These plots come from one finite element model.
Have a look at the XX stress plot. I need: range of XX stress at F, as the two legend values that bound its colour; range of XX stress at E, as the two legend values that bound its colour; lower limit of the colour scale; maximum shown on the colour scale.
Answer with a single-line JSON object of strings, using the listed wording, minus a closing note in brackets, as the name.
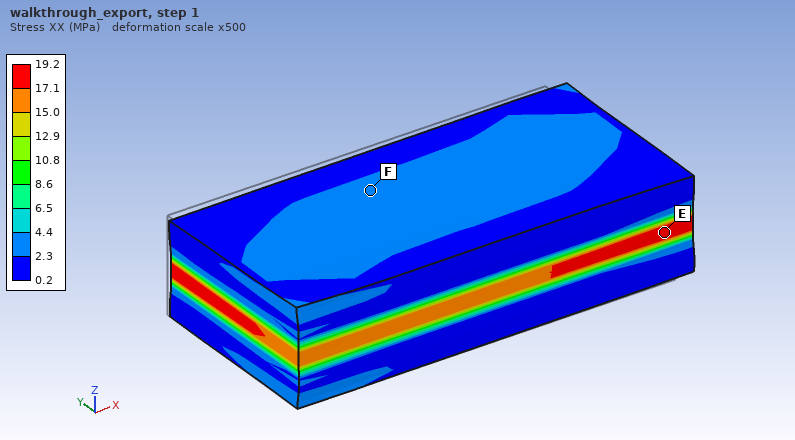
{"range of XX stress at F, as the two legend values that bound its colour": "2.3 to 4.4 MPa", "range of XX stress at E, as the two legend values that bound its colour": "17.1 to 19.2 MPa", "lower limit of the colour scale": "0.2 MPa", "maximum shown on the colour scale": "19.2 MPa"}
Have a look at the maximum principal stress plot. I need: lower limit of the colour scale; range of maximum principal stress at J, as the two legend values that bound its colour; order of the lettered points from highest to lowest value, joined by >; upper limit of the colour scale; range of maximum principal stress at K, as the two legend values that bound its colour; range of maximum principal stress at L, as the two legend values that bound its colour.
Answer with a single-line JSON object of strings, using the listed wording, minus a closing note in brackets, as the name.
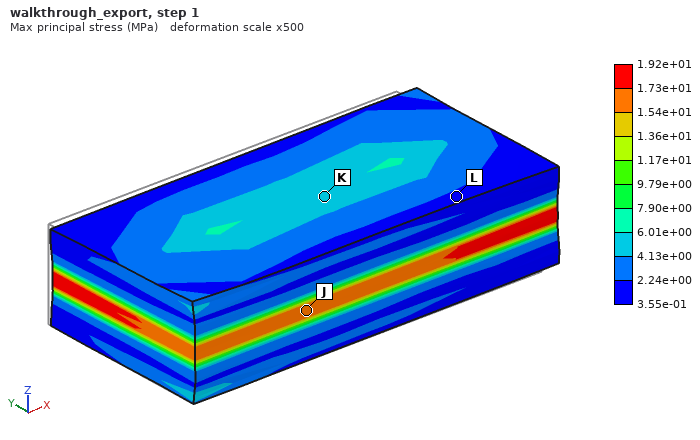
{"lower limit of the colour scale": "3.55e-01 MPa", "range of maximum principal stress at J, as the two legend values that bound its colour": "1.54e+01 to 1.73e+01 MPa", "order of the lettered points from highest to lowest value, joined by >": "J > K > L", "upper limit of the colour scale": "1.92e+01 MPa", "range of maximum principal stress at K, as the two legend values that bound its colour": "4.13e+00 to 6.01e+00 MPa", "range of maximum principal stress at L, as the two legend values that bound its colour": "3.55e-01 to 2.24e+00 MPa"}
